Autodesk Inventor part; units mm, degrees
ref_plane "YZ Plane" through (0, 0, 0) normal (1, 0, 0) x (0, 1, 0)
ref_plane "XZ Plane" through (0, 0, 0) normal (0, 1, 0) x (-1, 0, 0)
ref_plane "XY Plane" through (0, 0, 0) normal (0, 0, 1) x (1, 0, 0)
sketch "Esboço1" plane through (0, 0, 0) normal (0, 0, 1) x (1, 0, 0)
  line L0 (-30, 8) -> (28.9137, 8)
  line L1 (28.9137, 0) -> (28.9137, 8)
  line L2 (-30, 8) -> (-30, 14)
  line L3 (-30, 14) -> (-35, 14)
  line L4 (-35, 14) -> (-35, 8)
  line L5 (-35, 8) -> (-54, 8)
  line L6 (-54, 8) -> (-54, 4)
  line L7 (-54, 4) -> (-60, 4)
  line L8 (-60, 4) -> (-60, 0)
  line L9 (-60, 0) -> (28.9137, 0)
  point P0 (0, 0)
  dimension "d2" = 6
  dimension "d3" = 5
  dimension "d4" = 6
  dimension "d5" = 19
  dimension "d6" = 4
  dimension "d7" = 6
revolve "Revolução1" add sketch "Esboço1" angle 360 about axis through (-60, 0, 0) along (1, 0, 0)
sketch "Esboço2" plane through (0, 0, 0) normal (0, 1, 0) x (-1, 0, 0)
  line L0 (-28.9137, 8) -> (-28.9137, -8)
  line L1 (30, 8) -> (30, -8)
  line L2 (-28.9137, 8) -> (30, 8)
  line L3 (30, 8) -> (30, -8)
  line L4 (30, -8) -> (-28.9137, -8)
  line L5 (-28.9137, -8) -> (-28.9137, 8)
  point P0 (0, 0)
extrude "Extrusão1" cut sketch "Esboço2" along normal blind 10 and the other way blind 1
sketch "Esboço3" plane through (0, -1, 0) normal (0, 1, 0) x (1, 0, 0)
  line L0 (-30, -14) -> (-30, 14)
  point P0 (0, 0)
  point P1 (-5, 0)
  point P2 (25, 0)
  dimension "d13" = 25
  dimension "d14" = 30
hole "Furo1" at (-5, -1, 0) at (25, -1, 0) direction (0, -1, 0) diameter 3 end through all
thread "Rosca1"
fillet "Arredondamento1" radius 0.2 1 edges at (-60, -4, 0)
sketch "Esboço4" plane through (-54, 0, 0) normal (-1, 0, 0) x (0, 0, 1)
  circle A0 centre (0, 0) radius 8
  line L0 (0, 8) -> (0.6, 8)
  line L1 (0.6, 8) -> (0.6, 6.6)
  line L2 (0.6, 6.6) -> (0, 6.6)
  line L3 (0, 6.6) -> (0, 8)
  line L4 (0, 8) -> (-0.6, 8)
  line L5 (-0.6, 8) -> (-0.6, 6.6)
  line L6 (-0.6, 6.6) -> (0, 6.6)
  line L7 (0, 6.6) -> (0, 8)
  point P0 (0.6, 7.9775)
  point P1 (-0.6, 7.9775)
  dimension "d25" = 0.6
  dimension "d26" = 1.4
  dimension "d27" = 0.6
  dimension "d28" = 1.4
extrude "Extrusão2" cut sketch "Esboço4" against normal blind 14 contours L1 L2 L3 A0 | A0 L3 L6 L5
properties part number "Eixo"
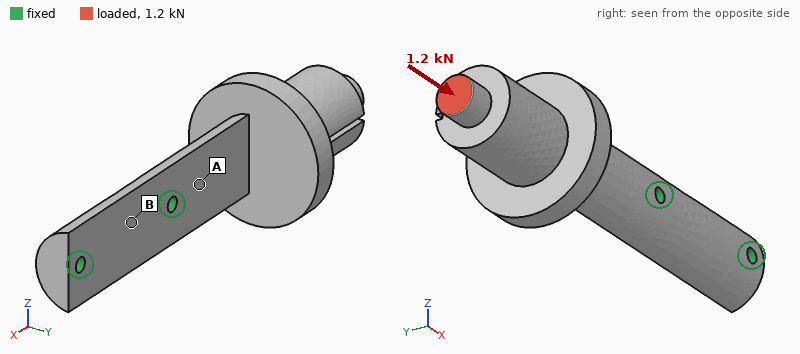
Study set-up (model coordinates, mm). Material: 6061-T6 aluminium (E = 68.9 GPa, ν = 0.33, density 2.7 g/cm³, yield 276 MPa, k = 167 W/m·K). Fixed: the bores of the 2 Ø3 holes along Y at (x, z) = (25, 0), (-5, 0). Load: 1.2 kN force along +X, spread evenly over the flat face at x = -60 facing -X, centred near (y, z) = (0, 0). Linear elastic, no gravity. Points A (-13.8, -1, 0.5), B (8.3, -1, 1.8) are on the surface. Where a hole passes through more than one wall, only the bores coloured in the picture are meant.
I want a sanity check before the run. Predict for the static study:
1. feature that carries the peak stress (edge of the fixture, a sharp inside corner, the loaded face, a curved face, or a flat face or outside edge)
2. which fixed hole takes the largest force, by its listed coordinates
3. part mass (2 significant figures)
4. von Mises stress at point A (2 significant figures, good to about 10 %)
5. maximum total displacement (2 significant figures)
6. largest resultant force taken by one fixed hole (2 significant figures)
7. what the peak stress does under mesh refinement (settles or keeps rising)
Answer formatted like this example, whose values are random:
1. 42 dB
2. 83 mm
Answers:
1. edge of the fixture
2. (-5, 0)
3. 33 g
4. 66 MPa
5. 0.28 mm
6. 1.1 kN
7. keeps rising
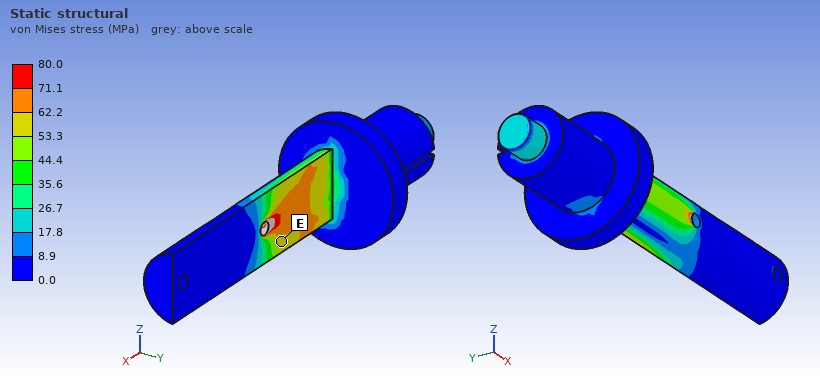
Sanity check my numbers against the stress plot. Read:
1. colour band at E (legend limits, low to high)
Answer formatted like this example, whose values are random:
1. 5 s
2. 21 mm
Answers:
1. 53.3 to 62.2 MPa
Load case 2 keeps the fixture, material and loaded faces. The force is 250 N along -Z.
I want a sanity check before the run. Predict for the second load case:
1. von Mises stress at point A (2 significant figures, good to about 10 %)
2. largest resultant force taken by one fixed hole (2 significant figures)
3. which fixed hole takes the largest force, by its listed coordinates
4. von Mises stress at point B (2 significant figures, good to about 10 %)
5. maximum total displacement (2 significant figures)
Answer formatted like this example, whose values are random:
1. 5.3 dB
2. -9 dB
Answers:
1. 22 MPa
2. 560 N
3. (-5, 0)
4. 11 MPa
5. 0.22 mm
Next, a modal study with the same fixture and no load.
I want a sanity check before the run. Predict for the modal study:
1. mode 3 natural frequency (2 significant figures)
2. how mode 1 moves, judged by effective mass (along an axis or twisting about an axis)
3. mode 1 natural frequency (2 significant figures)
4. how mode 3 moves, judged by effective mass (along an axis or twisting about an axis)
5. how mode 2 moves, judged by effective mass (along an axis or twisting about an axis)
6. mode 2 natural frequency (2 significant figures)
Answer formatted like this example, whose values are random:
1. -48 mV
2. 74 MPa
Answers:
1. 4300 Hz
2. along Y
3. 1200 Hz
4. twisting about X
5. along Z
6. 2000 Hz
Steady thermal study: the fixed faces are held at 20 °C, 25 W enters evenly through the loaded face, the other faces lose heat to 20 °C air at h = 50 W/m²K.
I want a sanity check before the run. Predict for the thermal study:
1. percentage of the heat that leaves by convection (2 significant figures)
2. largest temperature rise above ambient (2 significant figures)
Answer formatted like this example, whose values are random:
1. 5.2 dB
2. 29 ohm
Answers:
1. 26 %
2. 73 K
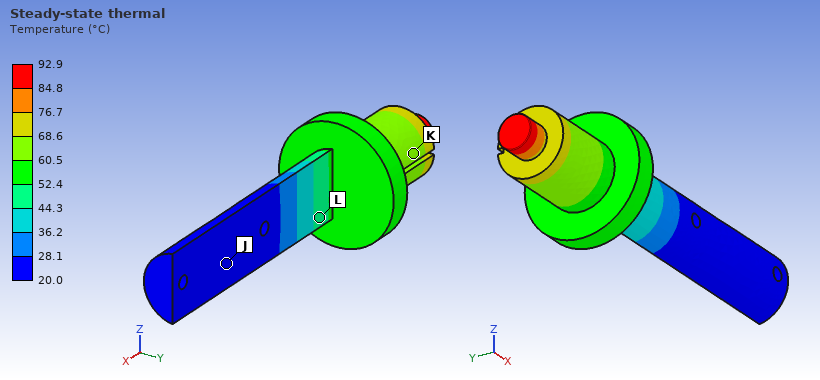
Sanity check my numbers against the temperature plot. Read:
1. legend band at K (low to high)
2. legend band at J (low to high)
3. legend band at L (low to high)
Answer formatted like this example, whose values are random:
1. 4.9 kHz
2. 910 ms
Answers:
1. 60.5 to 68.6 °C
2. 20.0 to 28.1 °C
3. 44.3 to 52.4 °C
